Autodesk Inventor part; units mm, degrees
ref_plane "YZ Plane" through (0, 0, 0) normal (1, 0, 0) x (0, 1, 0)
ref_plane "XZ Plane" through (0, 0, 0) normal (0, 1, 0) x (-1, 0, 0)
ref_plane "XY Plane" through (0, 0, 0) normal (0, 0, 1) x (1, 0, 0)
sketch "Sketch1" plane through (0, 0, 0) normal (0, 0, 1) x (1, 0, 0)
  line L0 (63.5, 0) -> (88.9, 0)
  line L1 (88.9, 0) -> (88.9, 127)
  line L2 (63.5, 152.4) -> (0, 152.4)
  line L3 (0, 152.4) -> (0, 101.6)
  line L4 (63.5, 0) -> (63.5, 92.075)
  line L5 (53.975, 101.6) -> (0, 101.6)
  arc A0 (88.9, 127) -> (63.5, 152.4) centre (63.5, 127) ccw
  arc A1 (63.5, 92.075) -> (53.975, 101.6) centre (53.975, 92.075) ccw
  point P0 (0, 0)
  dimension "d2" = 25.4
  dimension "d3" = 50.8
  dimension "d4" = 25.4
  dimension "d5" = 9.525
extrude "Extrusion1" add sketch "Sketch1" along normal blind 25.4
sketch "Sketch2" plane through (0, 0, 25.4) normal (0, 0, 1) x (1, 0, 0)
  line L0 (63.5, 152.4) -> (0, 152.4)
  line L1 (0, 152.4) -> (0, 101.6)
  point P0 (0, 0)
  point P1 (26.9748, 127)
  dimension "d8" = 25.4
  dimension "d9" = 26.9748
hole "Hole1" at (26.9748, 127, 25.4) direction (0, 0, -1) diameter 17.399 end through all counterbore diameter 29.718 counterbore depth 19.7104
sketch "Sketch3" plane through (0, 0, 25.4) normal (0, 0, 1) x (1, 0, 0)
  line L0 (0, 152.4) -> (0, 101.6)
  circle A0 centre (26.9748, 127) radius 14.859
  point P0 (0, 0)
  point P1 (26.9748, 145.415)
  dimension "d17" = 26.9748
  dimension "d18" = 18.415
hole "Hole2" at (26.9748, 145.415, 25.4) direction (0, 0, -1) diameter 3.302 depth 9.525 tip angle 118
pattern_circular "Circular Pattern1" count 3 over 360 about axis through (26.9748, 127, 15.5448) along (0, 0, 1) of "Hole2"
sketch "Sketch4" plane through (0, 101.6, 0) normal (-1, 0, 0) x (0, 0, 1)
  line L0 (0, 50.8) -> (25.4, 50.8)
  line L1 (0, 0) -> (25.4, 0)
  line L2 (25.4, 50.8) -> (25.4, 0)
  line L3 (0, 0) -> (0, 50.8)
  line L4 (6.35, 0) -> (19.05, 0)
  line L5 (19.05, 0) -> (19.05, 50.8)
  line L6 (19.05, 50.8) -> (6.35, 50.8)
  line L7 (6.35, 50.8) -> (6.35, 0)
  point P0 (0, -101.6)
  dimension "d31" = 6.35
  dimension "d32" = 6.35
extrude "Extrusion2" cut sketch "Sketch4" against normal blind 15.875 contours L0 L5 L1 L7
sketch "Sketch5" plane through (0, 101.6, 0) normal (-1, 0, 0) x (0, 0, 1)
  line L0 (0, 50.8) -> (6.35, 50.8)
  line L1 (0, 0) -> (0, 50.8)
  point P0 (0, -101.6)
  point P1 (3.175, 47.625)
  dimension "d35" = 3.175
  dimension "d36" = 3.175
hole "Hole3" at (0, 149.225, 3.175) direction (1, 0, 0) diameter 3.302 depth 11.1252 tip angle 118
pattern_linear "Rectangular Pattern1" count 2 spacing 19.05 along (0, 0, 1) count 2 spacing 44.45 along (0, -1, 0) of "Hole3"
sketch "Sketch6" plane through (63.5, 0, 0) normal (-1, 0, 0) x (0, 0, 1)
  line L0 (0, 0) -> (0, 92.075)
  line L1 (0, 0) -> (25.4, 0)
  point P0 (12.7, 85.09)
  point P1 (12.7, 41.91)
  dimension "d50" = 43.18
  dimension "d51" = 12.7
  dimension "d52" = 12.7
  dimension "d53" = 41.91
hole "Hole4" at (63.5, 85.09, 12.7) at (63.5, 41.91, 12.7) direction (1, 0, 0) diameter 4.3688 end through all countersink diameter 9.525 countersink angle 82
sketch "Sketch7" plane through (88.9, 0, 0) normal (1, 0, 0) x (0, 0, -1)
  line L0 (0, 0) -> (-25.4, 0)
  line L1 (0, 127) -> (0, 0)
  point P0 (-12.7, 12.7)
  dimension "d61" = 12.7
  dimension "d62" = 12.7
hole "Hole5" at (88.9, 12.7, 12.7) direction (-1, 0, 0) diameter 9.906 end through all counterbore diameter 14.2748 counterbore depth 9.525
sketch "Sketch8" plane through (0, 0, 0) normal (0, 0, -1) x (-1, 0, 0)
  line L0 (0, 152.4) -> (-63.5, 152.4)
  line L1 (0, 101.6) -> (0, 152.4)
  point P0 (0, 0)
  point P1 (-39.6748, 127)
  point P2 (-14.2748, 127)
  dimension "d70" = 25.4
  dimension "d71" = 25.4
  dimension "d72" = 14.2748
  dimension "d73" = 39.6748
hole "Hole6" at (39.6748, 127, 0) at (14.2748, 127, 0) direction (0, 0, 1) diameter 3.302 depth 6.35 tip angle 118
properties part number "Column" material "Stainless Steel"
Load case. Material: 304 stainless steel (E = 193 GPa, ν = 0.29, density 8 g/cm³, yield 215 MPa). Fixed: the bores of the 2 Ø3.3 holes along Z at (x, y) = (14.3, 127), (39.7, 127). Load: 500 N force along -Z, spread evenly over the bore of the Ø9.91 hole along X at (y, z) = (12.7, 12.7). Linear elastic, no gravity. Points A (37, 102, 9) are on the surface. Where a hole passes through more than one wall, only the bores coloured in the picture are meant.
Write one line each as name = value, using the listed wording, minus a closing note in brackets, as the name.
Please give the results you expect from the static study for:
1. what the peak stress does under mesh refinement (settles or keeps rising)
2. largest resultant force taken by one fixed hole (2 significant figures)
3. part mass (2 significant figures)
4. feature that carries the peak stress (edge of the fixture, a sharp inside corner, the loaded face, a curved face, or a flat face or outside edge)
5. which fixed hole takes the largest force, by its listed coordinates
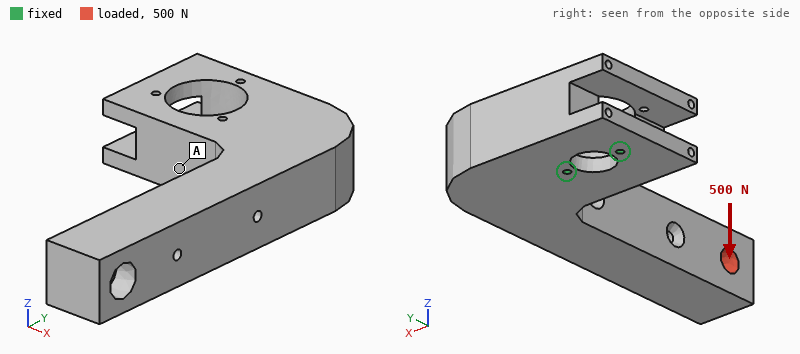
what the peak stress does under mesh refinement = keeps rising
largest resultant force taken by one fixed hole = 990 N
part mass = 1.2 kg
feature that carries the peak stress = edge of the fixture
which fixed hole takes the largest force, by its listed coordinates = (39.7, 127)
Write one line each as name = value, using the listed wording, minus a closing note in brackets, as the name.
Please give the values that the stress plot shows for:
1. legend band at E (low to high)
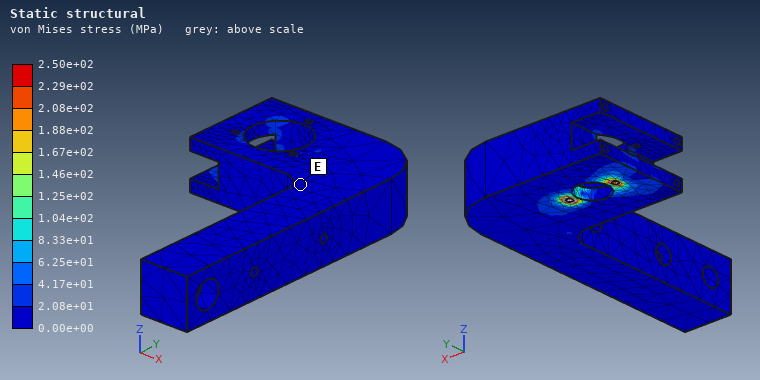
legend band at E = 0.00e+00 to 2.08e+01 MPa
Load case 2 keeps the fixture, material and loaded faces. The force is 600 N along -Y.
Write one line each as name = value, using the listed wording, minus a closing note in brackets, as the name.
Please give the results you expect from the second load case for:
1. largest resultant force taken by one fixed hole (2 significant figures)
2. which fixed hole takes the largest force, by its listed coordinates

largest resultant force taken by one fixed hole = 1.2 kN
which fixed hole takes the largest force, by its listed coordinates = (39.7, 127)
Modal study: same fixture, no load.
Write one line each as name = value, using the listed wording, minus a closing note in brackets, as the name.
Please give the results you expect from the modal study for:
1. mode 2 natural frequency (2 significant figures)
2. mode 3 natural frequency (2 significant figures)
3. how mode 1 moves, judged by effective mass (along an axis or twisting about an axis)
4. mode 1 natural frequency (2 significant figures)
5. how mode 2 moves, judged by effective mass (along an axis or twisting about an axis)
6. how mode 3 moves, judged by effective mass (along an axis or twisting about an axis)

mode 2 natural frequency = 960 Hz
mode 3 natural frequency = 1800 Hz
how mode 1 moves, judged by effective mass = along Z
mode 1 natural frequency = 400 Hz
how mode 2 moves, judged by effective mass = along X
how mode 3 moves, judged by effective mass = along Z
